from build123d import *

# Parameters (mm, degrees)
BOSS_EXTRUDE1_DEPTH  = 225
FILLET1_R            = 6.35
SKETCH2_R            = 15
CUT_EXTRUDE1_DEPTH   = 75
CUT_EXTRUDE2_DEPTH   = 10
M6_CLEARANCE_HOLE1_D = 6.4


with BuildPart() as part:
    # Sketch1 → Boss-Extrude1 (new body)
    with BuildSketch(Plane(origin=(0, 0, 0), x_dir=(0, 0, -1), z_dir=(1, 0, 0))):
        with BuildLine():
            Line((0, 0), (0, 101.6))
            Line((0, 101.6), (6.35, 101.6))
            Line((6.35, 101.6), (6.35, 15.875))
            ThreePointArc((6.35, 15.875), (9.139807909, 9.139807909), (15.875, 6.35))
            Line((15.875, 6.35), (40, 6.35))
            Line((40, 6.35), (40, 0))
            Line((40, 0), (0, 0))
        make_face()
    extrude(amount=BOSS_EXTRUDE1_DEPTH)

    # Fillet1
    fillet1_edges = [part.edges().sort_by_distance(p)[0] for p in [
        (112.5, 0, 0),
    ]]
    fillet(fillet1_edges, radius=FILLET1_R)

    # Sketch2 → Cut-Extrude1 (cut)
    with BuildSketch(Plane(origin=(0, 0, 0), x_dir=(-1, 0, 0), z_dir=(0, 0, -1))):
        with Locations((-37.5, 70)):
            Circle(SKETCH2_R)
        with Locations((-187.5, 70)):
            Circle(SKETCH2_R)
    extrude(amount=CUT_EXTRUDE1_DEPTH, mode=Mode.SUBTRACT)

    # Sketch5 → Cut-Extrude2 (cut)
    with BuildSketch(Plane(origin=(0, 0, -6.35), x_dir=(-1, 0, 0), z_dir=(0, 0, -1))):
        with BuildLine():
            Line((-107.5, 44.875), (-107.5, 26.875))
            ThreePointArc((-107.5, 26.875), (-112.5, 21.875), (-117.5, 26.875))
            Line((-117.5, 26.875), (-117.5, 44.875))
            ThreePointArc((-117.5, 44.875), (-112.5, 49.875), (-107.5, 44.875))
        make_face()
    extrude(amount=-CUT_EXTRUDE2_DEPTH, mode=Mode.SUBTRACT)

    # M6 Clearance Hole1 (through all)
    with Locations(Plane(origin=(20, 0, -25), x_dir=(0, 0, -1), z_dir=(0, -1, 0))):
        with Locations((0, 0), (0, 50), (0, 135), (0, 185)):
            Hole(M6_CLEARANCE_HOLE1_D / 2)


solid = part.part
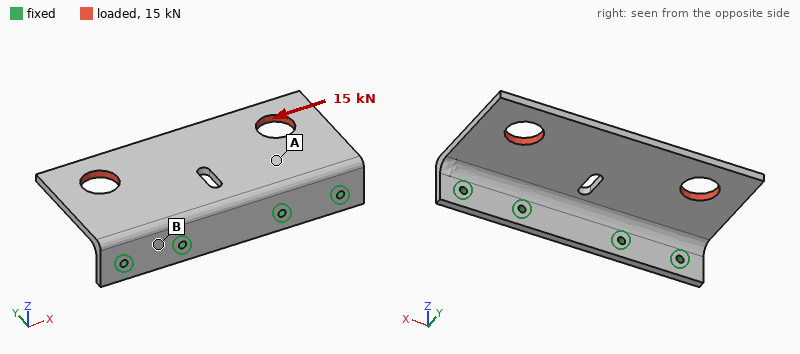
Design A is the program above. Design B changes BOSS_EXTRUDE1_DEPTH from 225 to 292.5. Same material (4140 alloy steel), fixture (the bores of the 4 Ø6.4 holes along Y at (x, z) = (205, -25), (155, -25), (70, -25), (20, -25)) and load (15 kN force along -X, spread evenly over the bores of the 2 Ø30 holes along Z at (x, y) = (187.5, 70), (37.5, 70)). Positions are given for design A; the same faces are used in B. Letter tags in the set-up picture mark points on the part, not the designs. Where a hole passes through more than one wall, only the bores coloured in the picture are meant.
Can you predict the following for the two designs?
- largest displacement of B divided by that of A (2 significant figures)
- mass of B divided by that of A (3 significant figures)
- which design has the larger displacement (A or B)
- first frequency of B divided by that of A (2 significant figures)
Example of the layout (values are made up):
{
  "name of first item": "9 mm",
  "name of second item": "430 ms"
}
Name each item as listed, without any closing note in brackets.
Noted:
{
  "largest displacement of B divided by that of A": "1.2",
  "mass of B divided by that of A": "1.32",
  "which design has the larger displacement": "B",
  "first frequency of B divided by that of A": "0.88"
}
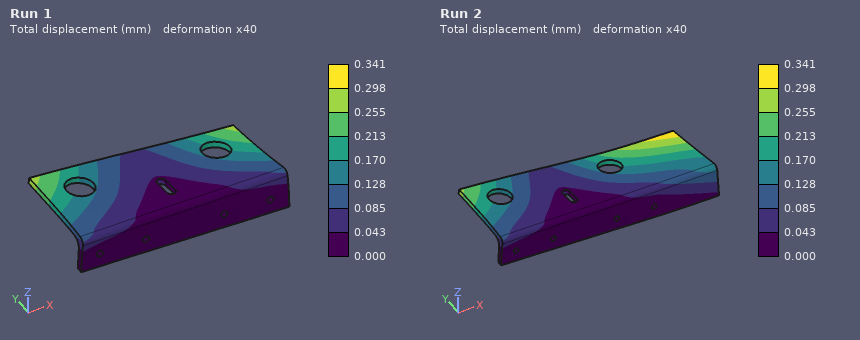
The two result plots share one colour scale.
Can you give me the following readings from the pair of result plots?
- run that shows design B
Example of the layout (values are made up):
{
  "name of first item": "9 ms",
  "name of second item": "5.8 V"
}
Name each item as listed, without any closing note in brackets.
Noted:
{
  "run that shows design B": "Run 2"
}
